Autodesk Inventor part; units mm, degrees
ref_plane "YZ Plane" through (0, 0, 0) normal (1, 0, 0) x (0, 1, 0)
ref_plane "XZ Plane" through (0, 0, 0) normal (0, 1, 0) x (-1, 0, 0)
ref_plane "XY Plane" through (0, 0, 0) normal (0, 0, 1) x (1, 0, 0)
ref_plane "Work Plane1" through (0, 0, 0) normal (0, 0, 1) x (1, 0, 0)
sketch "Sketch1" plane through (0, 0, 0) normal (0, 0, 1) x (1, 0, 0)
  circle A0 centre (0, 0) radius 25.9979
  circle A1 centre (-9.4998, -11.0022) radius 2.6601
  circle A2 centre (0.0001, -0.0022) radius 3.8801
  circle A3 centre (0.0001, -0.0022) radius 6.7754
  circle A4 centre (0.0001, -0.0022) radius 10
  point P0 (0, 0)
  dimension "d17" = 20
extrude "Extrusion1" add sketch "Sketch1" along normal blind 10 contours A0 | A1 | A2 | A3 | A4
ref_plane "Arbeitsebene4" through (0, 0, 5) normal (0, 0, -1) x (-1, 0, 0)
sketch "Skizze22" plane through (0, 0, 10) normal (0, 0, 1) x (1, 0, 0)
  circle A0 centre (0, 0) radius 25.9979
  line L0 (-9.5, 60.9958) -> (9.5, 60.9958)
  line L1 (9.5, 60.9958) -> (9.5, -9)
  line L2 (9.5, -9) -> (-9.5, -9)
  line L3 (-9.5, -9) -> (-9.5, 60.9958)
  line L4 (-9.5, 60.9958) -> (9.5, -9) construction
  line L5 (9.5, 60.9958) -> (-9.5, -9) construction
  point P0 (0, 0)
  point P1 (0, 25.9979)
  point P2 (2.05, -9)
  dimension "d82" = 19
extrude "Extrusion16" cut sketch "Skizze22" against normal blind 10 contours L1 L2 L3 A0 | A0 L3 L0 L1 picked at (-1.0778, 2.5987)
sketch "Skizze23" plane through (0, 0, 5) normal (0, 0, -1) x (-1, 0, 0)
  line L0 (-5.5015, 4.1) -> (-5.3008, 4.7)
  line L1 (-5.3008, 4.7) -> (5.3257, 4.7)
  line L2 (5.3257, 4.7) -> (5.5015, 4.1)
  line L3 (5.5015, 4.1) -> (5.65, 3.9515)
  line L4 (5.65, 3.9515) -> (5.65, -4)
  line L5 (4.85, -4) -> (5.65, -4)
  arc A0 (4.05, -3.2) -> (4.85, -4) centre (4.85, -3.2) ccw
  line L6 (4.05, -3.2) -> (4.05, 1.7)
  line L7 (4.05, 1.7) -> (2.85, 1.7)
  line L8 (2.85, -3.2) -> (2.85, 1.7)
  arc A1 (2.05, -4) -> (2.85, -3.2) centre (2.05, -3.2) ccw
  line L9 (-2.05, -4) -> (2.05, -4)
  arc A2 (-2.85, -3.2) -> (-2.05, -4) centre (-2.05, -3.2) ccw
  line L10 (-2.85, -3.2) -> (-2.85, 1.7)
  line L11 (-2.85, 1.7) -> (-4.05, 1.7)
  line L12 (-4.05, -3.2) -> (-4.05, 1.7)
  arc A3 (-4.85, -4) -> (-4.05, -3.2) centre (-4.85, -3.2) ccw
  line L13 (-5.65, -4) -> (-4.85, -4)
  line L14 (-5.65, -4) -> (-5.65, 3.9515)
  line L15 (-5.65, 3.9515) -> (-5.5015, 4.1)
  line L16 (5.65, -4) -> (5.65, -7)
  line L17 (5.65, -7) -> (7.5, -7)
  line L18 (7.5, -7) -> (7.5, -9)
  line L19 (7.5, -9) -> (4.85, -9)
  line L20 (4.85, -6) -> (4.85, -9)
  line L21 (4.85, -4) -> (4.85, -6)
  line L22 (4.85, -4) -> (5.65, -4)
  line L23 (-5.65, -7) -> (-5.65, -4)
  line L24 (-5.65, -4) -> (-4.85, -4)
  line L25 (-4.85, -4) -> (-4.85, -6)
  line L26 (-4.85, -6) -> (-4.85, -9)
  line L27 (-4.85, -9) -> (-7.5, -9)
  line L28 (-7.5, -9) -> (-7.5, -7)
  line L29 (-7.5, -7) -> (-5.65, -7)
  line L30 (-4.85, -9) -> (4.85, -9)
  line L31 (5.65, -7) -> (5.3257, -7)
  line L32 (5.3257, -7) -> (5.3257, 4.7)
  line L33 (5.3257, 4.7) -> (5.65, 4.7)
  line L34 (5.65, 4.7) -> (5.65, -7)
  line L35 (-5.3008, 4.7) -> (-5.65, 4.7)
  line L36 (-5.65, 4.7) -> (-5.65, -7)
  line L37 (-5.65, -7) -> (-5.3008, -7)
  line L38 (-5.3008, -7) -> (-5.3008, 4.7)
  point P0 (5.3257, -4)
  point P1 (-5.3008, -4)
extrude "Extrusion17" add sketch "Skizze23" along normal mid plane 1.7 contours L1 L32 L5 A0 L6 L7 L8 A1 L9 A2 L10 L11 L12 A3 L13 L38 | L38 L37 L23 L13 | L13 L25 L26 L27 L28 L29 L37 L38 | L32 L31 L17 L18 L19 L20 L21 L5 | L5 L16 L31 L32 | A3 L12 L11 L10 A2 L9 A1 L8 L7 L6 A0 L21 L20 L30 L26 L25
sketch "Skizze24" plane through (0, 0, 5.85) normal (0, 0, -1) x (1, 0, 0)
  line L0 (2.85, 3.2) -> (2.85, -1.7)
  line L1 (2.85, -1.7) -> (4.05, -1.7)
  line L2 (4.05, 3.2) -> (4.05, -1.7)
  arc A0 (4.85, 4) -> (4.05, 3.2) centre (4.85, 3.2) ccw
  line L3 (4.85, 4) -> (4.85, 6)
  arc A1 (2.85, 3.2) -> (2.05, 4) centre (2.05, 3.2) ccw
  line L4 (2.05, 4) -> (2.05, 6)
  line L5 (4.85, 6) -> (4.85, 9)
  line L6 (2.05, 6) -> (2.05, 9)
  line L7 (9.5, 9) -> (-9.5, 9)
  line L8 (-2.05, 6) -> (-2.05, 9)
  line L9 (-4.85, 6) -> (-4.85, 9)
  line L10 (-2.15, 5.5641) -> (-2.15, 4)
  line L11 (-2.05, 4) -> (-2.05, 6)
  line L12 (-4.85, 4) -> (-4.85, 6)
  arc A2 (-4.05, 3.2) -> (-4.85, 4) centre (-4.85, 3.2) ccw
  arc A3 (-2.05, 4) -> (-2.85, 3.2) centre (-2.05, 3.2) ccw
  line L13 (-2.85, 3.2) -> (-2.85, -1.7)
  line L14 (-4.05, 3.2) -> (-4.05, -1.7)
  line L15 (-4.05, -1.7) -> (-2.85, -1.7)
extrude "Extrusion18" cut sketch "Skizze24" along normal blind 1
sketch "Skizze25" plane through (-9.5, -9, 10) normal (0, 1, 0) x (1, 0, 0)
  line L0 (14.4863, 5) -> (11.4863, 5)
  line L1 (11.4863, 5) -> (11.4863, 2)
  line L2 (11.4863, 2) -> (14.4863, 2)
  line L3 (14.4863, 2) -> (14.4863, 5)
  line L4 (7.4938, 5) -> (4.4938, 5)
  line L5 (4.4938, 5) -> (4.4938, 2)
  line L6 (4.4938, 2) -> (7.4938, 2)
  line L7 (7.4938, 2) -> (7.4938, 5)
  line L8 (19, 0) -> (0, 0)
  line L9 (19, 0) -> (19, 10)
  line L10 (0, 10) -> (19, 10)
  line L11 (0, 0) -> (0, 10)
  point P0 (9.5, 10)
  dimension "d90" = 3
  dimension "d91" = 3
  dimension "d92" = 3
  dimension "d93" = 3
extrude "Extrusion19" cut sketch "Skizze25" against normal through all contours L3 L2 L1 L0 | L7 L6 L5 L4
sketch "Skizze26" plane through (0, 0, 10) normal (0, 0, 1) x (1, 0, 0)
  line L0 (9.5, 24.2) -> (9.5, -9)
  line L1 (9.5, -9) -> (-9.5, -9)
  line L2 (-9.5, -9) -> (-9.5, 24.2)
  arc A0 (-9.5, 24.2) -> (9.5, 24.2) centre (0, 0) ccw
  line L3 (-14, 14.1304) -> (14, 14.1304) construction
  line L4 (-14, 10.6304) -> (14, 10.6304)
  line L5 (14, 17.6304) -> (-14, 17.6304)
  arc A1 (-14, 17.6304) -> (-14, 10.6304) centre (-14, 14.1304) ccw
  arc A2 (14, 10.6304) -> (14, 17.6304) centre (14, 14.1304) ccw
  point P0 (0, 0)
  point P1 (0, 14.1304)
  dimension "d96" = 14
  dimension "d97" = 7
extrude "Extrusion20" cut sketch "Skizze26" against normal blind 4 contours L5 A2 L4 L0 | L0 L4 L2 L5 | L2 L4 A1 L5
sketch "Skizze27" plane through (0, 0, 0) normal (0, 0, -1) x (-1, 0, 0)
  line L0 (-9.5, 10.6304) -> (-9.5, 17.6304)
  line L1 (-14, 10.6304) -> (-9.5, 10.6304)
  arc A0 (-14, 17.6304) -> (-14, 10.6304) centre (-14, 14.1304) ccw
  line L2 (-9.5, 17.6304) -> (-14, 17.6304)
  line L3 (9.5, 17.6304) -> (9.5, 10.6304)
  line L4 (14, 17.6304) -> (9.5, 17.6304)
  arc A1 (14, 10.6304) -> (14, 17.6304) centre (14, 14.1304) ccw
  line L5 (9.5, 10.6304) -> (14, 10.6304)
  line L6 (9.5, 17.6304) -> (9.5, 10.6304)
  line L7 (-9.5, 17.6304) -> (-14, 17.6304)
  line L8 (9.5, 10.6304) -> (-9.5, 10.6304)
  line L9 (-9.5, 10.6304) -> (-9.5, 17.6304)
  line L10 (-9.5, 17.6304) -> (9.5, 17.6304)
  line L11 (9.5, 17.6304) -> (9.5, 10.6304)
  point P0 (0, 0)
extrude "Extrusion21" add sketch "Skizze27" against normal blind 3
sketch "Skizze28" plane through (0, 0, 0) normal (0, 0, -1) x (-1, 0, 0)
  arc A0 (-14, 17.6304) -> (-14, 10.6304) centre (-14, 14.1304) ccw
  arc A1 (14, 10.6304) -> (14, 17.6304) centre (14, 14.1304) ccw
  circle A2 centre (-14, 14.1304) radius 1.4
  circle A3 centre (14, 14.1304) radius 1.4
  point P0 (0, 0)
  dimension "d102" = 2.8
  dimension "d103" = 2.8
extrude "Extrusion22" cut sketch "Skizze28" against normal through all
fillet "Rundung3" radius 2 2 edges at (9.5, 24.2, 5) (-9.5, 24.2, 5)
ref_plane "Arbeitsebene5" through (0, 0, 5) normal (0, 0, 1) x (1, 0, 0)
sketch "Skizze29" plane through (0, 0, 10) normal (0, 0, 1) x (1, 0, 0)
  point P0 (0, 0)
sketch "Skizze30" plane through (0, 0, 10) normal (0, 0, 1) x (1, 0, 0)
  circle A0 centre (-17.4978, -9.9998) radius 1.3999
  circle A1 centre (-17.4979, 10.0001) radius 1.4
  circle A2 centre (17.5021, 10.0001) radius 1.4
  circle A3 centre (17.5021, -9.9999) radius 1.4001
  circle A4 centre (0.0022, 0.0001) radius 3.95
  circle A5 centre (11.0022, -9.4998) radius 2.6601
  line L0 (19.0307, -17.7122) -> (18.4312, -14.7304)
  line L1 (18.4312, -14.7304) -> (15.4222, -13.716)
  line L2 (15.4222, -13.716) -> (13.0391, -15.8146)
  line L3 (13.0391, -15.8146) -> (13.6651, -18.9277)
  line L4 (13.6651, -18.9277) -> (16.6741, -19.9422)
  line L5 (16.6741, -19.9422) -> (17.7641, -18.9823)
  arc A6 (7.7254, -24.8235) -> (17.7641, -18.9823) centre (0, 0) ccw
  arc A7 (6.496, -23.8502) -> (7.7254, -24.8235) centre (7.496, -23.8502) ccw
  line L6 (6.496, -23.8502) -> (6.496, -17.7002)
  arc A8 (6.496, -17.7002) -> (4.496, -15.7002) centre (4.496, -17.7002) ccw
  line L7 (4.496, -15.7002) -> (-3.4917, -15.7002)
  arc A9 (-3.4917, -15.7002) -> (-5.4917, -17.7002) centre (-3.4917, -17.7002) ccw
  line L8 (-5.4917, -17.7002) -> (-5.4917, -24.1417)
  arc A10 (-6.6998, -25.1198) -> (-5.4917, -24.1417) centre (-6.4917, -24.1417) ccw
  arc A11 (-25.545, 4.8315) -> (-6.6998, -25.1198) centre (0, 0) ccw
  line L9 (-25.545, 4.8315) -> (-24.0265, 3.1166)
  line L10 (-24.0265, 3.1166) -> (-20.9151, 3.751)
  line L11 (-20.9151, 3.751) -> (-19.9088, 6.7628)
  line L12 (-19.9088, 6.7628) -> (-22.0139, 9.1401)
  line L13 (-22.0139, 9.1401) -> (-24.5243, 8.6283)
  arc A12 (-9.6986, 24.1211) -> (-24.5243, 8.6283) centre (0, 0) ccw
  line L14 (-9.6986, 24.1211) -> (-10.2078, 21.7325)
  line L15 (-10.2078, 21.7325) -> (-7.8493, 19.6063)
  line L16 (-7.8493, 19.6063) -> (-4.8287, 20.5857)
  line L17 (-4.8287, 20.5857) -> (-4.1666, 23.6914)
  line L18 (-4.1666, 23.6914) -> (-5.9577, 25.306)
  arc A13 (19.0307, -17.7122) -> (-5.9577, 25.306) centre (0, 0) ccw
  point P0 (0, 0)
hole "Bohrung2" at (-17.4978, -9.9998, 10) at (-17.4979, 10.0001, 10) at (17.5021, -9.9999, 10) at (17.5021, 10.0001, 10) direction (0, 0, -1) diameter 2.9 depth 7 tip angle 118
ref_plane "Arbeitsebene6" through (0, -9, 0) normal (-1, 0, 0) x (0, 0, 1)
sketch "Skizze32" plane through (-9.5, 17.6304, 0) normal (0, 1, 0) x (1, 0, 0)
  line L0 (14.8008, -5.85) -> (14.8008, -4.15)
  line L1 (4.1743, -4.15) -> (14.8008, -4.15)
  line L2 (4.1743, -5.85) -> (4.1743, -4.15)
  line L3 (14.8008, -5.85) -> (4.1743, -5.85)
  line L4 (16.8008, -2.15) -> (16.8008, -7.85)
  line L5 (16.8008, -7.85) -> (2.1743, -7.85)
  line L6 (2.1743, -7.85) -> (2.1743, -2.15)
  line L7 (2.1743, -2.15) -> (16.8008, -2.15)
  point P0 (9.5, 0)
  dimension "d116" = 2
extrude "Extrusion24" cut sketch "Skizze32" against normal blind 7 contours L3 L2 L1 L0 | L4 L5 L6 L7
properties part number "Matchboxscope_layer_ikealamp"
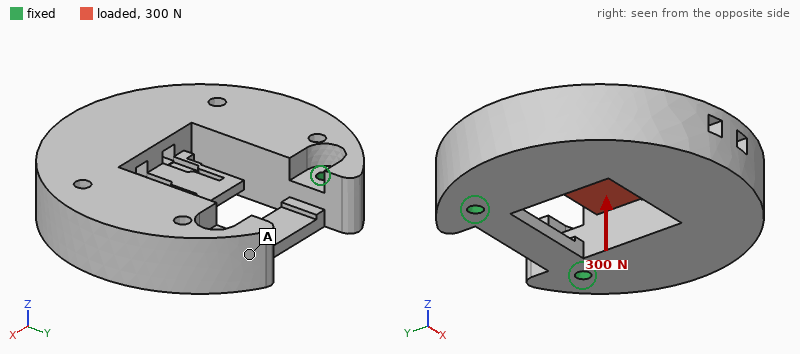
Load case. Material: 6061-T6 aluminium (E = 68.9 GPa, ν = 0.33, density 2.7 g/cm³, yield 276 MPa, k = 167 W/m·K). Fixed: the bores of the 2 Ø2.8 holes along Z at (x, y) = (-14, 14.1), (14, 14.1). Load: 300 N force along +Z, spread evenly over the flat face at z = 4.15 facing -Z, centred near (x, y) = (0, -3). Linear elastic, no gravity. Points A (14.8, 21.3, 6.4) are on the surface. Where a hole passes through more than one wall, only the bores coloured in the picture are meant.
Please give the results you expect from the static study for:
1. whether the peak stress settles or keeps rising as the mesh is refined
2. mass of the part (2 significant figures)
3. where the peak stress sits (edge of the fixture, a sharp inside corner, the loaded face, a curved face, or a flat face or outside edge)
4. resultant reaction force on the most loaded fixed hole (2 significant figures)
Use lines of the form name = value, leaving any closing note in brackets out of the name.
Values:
whether the peak stress settles or keeps rising as the mesh is refined = keeps rising
mass of the part = 38 g
where the peak stress sits = a sharp inside corner
resultant reaction force on the most loaded fixed hole = 150 N
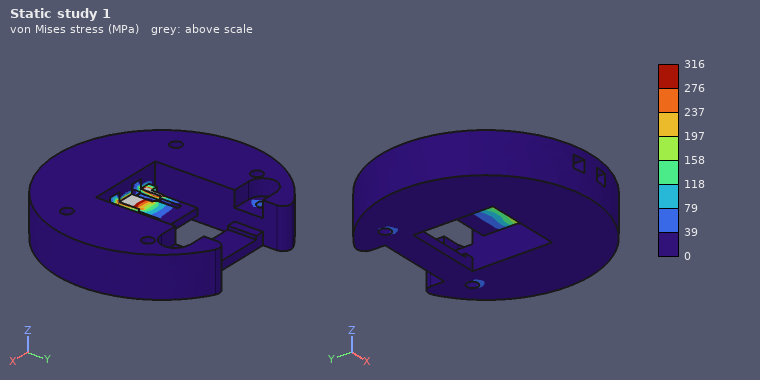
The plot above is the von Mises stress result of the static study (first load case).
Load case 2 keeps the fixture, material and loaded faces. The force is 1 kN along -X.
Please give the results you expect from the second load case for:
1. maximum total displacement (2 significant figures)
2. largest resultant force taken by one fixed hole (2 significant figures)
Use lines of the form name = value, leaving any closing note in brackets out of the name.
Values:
maximum total displacement = 0.11 mm
largest resultant force taken by one fixed hole = 600 N
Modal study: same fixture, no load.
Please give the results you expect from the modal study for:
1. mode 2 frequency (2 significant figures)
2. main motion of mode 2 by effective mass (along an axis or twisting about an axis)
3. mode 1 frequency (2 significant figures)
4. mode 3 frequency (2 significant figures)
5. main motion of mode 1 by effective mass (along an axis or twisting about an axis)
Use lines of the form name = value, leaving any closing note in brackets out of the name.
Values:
mode 2 frequency = 5600 Hz
main motion of mode 2 by effective mass = along X
mode 1 frequency = 2900 Hz
mode 3 frequency = 6200 Hz
main motion of mode 1 by effective mass = along Z
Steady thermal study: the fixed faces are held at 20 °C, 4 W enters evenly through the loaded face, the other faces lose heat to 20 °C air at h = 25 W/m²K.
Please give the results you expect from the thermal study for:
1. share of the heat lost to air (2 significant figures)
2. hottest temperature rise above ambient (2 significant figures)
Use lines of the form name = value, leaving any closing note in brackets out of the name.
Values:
share of the heat lost to air = 8.5 %
hottest temperature rise above ambient = 15 K
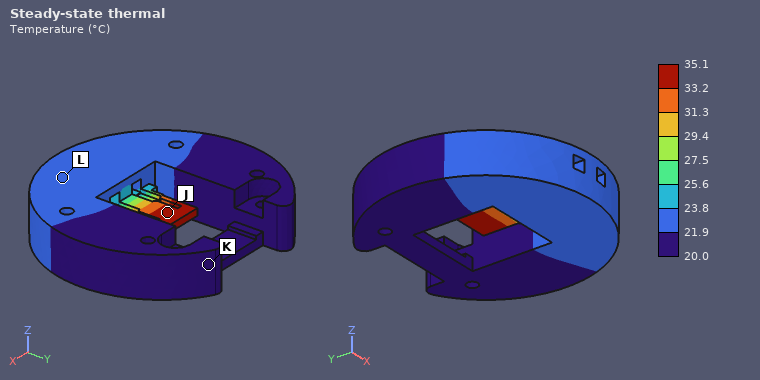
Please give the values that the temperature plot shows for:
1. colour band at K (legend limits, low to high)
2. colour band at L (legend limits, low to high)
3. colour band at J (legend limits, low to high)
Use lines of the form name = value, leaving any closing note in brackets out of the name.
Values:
colour band at K = 20.0 to 21.9 °C
colour band at L = 21.9 to 23.8 °C
colour band at J = 33.2 to 35.1 °C
